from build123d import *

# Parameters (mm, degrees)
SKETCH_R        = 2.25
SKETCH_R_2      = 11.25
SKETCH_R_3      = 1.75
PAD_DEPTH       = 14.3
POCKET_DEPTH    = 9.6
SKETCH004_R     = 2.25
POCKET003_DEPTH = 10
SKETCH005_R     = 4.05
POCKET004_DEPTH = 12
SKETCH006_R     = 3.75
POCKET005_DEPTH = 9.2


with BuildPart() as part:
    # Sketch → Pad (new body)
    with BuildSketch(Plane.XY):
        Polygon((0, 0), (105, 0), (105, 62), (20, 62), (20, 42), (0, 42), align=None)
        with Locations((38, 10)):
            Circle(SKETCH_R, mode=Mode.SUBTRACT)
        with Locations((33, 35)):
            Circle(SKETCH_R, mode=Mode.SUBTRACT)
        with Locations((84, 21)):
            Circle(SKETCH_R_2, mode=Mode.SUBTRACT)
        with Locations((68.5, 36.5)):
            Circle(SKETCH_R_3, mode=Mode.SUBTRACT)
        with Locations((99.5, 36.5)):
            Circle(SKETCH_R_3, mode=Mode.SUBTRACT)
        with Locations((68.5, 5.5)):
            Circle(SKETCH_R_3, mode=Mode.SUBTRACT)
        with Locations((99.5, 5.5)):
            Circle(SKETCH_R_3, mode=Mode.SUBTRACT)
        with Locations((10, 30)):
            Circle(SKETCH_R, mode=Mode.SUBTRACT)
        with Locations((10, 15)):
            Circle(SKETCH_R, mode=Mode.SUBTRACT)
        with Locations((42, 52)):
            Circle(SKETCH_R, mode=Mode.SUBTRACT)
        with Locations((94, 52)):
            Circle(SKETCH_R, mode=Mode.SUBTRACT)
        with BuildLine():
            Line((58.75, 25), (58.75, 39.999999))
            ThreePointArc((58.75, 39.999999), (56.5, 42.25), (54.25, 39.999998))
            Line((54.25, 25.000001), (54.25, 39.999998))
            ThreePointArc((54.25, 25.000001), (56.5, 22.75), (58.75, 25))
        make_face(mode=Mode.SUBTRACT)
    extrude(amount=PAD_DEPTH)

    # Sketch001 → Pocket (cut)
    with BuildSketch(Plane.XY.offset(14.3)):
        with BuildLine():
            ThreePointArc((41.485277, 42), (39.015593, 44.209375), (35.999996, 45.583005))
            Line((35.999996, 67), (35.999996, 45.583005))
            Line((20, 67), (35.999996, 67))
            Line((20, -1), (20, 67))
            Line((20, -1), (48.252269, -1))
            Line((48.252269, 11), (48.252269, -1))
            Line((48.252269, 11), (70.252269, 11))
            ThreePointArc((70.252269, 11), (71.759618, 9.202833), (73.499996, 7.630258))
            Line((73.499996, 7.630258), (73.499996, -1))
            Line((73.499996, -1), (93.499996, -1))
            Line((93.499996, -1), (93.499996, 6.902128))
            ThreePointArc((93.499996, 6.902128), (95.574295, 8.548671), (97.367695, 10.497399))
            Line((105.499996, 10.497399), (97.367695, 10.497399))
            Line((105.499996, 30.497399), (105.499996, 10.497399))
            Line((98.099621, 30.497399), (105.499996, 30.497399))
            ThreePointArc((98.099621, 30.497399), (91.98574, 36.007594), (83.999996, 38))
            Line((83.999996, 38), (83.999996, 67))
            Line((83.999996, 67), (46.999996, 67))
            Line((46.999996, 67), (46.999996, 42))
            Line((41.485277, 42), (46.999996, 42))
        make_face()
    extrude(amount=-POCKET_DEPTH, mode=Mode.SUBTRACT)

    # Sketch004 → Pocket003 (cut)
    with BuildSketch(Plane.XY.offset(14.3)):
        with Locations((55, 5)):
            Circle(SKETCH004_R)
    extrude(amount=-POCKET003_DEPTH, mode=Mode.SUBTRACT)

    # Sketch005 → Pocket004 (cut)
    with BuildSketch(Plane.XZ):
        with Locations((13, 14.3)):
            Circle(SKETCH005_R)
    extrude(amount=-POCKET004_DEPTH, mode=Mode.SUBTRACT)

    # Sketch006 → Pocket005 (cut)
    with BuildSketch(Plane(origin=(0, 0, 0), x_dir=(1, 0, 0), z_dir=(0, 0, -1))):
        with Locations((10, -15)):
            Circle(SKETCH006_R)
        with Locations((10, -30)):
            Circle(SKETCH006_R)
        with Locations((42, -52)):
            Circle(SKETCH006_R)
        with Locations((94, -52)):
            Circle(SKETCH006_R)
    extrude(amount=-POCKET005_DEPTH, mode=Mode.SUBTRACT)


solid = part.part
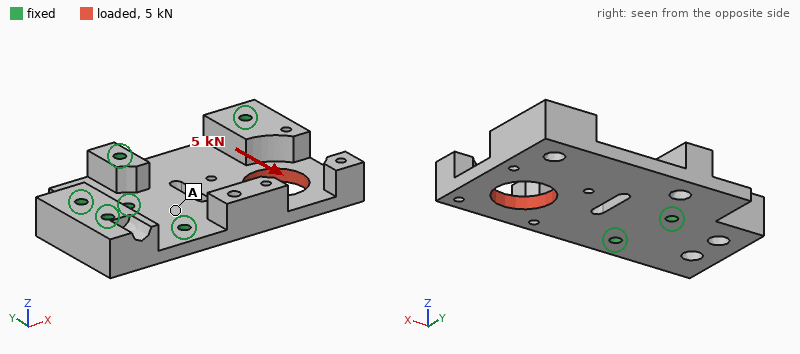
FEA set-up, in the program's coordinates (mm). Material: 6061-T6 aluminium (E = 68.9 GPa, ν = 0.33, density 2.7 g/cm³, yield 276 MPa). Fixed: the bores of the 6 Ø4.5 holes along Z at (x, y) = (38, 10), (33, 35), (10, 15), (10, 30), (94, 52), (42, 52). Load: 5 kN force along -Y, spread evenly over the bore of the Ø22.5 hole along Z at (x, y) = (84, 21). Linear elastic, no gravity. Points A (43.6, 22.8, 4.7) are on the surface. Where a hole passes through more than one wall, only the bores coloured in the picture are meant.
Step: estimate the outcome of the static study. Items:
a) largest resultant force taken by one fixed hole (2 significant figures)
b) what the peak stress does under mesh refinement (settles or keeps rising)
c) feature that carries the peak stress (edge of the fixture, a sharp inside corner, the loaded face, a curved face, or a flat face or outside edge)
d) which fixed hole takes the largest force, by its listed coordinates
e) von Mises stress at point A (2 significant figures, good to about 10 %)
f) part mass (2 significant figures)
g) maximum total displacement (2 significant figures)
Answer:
2.7 kN
keeps rising
edge of the fixture
(94, 52)
19 MPa
120 g
0.14 mm
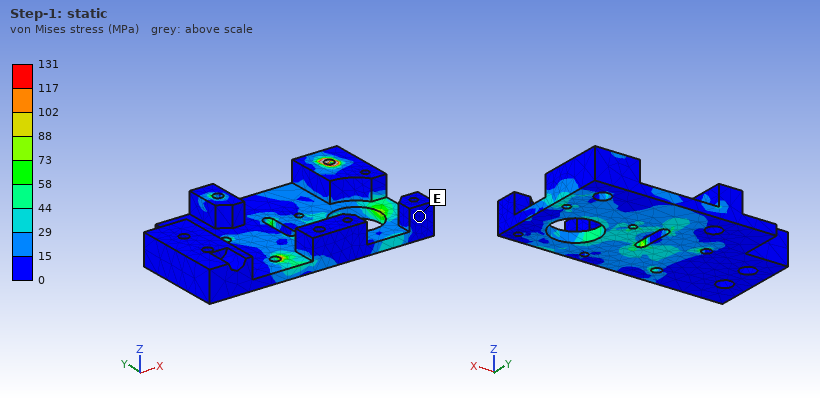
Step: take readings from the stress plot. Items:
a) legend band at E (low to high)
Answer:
0 to 15 MPa
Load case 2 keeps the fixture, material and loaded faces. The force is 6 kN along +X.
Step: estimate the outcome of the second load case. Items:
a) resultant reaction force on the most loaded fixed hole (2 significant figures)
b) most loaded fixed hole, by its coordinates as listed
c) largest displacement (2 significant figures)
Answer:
2.9 kN
(38, 10)
42 µm
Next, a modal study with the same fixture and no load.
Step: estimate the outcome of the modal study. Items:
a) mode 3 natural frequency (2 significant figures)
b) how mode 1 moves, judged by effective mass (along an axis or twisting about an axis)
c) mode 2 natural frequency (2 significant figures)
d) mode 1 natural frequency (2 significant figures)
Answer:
6500 Hz
along Z
5100 Hz
2300 Hz
